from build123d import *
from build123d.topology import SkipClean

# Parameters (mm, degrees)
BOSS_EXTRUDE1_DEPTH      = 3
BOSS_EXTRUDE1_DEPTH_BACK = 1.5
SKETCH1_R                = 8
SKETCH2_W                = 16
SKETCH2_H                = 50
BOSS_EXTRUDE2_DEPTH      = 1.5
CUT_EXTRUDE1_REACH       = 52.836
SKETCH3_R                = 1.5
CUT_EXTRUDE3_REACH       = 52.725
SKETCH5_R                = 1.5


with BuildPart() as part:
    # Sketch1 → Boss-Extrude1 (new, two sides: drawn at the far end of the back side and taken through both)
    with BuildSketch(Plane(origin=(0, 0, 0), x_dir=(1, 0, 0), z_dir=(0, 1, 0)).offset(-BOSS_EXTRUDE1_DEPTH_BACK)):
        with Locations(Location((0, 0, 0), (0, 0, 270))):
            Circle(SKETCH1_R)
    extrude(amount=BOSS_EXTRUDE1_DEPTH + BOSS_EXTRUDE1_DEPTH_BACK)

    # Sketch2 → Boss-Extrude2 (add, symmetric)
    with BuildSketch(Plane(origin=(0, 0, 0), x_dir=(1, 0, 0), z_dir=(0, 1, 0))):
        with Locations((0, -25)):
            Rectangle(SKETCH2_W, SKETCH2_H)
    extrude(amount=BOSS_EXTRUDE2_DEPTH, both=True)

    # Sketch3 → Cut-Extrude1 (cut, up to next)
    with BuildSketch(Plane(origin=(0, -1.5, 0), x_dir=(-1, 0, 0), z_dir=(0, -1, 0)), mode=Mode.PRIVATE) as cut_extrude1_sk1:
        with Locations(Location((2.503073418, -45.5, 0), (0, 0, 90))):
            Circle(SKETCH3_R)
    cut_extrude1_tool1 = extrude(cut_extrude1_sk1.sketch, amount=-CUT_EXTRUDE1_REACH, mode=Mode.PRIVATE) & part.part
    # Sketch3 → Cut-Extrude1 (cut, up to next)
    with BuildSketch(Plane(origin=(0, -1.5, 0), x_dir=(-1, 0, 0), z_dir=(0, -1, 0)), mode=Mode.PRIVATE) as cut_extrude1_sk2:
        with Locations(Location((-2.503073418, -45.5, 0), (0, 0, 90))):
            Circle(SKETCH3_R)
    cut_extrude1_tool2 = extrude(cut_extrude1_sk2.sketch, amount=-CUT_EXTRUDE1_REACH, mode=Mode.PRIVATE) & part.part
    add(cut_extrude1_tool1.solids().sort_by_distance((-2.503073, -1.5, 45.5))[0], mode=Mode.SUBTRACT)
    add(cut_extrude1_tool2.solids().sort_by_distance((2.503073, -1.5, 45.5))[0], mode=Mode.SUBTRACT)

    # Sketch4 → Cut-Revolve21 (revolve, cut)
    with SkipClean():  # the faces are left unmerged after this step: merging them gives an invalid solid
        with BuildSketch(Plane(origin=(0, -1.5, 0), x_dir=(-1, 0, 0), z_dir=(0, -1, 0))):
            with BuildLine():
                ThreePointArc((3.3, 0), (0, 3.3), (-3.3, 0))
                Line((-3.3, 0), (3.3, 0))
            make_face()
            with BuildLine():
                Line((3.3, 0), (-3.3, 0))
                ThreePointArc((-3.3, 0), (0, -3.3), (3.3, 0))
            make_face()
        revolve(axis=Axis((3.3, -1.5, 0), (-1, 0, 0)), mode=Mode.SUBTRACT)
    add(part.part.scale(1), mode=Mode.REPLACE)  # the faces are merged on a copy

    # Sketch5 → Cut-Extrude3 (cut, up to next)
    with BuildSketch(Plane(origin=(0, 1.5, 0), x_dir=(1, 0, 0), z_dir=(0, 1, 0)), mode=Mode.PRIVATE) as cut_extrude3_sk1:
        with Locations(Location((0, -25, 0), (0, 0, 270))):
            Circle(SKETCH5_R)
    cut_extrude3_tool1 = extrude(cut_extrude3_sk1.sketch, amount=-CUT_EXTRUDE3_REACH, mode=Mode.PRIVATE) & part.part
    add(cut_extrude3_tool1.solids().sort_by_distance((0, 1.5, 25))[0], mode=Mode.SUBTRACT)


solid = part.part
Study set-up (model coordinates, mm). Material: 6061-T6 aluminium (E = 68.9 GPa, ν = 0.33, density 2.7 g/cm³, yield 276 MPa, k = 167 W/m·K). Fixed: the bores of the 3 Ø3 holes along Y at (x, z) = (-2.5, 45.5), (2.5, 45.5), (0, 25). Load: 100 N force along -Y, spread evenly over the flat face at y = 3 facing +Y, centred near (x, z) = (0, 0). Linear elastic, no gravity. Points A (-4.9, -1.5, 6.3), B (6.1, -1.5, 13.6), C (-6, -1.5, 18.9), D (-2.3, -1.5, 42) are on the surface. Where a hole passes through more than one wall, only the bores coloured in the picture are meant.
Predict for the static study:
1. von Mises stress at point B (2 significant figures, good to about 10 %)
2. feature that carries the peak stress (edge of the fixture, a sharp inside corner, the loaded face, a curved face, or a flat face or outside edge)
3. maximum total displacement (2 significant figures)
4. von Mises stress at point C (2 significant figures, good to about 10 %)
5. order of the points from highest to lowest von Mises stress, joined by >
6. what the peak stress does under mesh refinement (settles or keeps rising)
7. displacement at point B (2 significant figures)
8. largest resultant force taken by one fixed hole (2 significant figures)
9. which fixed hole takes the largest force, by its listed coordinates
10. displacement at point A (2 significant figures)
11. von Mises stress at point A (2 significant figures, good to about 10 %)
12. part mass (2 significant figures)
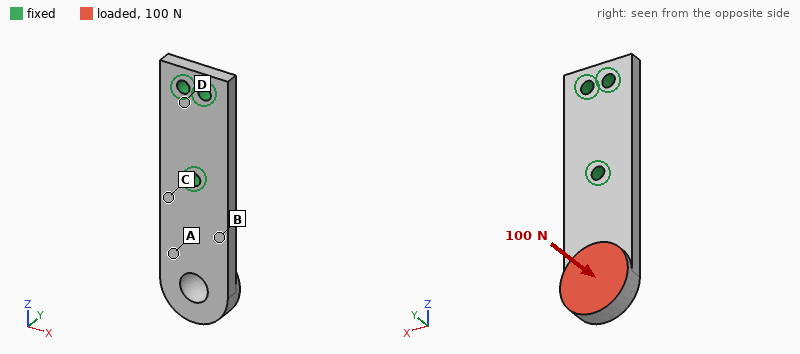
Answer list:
56 MPa
edge of the fixture
0.30 mm
74 MPa
C > B > A > D
keeps rising
0.057 mm
130 N
(0, 25)
0.13 mm
22 MPa
7.7 g
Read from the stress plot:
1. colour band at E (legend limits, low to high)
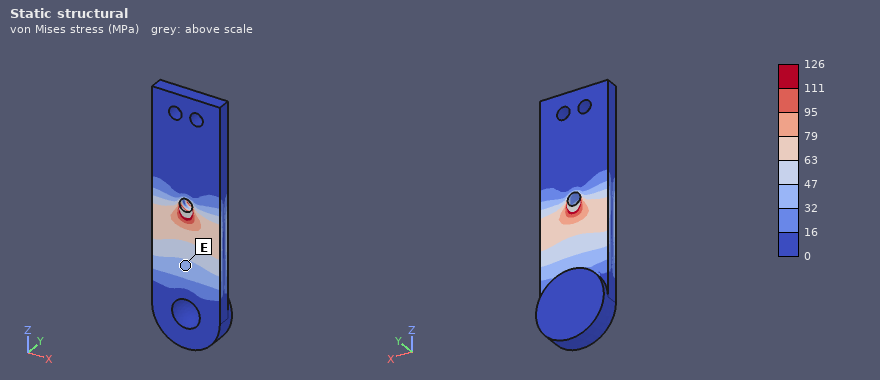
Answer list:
32 to 47 MPa
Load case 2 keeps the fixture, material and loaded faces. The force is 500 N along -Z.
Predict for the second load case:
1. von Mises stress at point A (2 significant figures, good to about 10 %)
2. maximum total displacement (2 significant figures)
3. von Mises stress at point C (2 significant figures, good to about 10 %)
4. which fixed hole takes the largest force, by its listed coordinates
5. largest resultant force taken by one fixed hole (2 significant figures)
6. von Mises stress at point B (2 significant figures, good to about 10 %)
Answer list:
35 MPa
0.28 mm
51 MPa
(0, 25)
420 N
53 MPa
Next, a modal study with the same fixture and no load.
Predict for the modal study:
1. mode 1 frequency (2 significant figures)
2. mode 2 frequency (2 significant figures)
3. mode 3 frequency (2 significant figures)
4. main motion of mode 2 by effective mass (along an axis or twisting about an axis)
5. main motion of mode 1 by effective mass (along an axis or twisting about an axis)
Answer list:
2200 Hz
7300 Hz
8500 Hz
along X
along Y
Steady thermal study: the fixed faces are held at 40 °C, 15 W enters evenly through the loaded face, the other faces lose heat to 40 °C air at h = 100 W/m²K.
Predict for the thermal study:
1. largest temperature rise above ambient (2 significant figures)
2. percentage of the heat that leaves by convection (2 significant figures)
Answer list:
41 K
19 %
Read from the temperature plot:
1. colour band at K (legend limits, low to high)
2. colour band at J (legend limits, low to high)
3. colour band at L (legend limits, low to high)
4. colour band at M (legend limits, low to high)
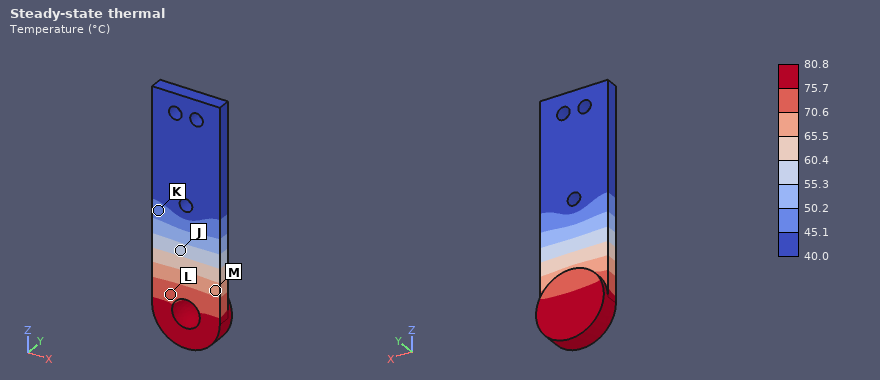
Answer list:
45.1 to 50.2 °C
55.3 to 60.4 °C
70.6 to 75.7 °C
65.5 to 70.6 °C
